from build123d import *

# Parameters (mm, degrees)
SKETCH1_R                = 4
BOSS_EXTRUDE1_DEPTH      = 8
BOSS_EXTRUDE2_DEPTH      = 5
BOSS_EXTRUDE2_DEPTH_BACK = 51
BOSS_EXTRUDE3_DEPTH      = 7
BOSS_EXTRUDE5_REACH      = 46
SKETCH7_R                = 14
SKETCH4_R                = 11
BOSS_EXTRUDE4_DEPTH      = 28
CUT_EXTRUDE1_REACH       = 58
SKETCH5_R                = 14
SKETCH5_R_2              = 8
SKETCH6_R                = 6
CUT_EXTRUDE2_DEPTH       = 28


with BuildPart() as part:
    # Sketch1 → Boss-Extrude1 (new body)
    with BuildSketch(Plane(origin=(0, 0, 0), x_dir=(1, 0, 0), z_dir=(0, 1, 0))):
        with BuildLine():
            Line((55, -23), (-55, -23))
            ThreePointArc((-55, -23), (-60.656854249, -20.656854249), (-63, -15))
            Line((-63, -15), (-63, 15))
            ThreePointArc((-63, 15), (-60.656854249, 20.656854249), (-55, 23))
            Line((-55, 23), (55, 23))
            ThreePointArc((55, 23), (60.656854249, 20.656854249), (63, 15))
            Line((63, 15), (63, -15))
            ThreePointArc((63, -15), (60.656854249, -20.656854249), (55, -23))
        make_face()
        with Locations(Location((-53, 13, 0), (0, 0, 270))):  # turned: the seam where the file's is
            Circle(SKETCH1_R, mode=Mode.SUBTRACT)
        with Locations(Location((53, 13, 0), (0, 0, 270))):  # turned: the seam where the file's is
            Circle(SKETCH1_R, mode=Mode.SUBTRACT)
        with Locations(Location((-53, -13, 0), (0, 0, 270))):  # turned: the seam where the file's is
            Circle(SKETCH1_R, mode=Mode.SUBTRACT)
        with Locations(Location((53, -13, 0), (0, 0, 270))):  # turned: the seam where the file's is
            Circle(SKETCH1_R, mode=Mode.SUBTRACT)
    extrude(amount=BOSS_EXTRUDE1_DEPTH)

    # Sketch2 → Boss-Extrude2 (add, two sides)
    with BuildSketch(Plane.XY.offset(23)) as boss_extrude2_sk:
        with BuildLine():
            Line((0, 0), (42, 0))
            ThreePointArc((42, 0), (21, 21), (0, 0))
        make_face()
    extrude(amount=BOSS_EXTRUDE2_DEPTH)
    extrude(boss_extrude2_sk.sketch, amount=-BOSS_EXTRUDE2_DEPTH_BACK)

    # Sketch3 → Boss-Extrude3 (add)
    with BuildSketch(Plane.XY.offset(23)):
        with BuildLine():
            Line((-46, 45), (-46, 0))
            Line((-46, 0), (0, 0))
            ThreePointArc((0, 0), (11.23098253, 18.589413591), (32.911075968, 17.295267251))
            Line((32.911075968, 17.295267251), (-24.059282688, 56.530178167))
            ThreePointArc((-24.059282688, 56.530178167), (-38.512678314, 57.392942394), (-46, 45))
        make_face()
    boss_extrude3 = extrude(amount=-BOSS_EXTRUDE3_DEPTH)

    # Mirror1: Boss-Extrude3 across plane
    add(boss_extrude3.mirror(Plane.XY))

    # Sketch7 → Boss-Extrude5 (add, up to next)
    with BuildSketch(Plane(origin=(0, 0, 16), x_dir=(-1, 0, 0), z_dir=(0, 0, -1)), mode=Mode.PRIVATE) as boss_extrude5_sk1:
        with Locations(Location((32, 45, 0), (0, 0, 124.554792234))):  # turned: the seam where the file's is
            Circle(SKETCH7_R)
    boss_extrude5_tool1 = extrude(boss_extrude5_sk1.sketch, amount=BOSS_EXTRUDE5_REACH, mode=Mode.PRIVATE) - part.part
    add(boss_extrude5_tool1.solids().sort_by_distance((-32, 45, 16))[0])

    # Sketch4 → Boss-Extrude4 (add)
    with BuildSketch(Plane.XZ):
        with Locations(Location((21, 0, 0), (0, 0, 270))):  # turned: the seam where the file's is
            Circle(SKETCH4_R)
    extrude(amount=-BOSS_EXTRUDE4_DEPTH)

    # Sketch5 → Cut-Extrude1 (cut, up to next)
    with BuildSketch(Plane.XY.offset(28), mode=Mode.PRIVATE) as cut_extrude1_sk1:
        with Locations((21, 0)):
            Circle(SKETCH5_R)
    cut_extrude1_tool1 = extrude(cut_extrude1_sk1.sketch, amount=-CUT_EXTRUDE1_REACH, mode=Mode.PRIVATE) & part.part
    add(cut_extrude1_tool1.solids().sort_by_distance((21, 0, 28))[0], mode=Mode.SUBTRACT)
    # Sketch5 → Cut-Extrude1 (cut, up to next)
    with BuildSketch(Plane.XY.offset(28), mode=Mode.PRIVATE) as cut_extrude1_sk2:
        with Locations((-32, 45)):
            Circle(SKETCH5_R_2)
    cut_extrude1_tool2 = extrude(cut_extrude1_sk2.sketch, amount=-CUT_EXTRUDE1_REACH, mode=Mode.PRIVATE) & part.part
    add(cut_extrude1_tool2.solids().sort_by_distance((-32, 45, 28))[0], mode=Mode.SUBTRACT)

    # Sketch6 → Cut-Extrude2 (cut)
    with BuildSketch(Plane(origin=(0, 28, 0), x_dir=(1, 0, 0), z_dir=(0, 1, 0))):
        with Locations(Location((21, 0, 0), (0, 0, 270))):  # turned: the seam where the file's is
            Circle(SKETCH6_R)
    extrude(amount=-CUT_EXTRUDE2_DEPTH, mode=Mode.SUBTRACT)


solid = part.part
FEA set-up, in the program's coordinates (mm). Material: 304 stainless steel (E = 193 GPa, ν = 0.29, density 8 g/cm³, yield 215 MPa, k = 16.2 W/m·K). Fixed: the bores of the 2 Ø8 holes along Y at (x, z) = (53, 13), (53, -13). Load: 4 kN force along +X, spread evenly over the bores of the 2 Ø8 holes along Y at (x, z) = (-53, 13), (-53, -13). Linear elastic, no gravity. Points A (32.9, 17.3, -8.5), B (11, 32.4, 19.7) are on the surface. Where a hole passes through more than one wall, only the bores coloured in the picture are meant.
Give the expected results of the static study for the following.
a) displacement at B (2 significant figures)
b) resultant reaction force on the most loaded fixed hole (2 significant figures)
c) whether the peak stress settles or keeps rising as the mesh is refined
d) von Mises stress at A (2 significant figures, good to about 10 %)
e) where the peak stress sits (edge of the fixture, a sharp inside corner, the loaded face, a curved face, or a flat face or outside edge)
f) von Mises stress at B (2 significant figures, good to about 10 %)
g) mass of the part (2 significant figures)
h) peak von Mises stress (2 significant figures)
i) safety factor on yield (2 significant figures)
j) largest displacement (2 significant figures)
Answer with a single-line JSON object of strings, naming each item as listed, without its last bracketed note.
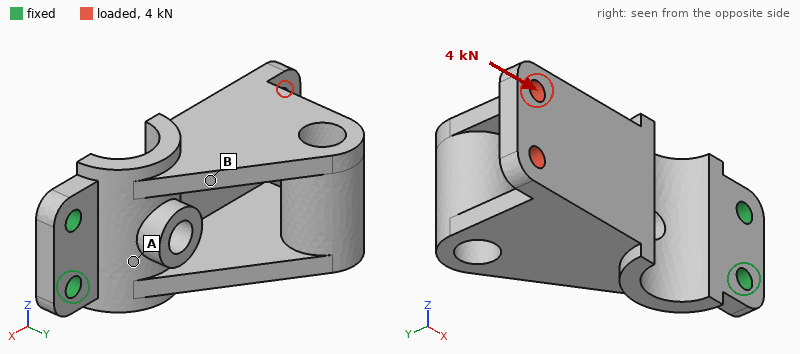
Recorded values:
{"displacement at B": "0.068 mm", "resultant reaction force on the most loaded fixed hole": "2.0 kN", "whether the peak stress settles or keeps rising as the mesh is refined": "settles", "von Mises stress at A": "58 MPa", "where the peak stress sits": "a curved face", "von Mises stress at B": "21 MPa", "mass of the part": "770 g", "peak von Mises stress": "180 MPa", "safety factor on yield": "1.2", "largest displacement": "0.29 mm"}
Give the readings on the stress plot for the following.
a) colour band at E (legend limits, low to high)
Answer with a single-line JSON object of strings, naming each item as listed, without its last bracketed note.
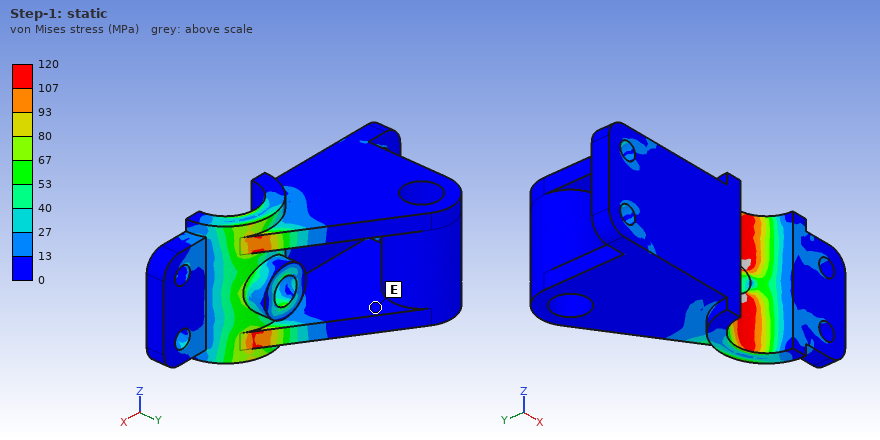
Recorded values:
{"colour band at E": "0 to 13 MPa"}
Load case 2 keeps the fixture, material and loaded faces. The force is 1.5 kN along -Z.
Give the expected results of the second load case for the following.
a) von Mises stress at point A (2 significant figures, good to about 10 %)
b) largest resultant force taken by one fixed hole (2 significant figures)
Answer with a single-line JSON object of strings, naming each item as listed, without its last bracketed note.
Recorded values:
{"von Mises stress at point A": "65 MPa", "largest resultant force taken by one fixed hole": "5.1 kN"}
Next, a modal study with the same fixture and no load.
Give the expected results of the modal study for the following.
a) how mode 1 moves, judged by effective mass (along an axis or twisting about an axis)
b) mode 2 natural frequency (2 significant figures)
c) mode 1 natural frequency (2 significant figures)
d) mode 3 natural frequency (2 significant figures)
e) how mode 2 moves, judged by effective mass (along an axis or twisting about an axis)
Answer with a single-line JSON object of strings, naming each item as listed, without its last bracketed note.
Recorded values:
{"how mode 1 moves, judged by effective mass": "along Y", "mode 2 natural frequency": "1100 Hz", "mode 1 natural frequency": "310 Hz", "mode 3 natural frequency": "1500 Hz", "how mode 2 moves, judged by effective mass": "along Z"}
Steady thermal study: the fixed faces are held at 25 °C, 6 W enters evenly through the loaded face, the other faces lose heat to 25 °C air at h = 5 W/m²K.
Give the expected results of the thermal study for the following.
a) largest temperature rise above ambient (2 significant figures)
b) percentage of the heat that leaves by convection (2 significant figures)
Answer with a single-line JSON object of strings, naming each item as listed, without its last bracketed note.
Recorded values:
{"largest temperature rise above ambient": "55 K", "percentage of the heat that leaves by convection": "59 %"}
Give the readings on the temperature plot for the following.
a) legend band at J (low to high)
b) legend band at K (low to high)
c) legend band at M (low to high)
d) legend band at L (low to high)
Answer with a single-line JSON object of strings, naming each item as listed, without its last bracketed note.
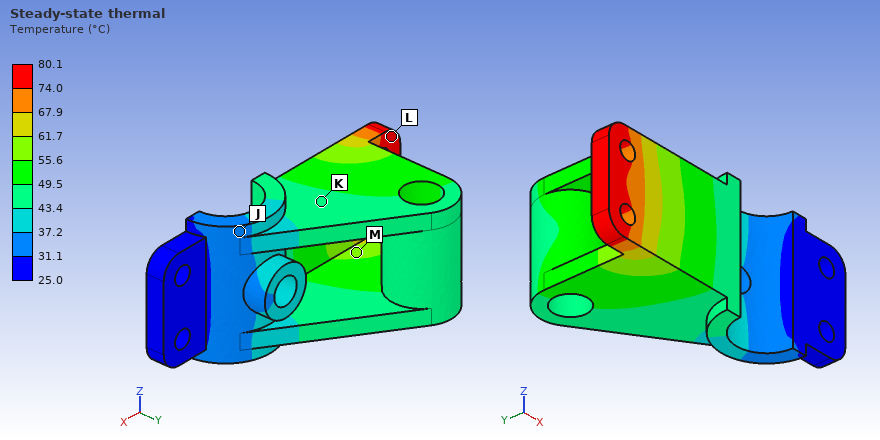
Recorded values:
{"legend band at J": "31.1 to 37.2 °C", "legend band at K": "43.4 to 49.5 °C", "legend band at M": "55.6 to 61.7 °C", "legend band at L": "74.0 to 80.1 °C"}
